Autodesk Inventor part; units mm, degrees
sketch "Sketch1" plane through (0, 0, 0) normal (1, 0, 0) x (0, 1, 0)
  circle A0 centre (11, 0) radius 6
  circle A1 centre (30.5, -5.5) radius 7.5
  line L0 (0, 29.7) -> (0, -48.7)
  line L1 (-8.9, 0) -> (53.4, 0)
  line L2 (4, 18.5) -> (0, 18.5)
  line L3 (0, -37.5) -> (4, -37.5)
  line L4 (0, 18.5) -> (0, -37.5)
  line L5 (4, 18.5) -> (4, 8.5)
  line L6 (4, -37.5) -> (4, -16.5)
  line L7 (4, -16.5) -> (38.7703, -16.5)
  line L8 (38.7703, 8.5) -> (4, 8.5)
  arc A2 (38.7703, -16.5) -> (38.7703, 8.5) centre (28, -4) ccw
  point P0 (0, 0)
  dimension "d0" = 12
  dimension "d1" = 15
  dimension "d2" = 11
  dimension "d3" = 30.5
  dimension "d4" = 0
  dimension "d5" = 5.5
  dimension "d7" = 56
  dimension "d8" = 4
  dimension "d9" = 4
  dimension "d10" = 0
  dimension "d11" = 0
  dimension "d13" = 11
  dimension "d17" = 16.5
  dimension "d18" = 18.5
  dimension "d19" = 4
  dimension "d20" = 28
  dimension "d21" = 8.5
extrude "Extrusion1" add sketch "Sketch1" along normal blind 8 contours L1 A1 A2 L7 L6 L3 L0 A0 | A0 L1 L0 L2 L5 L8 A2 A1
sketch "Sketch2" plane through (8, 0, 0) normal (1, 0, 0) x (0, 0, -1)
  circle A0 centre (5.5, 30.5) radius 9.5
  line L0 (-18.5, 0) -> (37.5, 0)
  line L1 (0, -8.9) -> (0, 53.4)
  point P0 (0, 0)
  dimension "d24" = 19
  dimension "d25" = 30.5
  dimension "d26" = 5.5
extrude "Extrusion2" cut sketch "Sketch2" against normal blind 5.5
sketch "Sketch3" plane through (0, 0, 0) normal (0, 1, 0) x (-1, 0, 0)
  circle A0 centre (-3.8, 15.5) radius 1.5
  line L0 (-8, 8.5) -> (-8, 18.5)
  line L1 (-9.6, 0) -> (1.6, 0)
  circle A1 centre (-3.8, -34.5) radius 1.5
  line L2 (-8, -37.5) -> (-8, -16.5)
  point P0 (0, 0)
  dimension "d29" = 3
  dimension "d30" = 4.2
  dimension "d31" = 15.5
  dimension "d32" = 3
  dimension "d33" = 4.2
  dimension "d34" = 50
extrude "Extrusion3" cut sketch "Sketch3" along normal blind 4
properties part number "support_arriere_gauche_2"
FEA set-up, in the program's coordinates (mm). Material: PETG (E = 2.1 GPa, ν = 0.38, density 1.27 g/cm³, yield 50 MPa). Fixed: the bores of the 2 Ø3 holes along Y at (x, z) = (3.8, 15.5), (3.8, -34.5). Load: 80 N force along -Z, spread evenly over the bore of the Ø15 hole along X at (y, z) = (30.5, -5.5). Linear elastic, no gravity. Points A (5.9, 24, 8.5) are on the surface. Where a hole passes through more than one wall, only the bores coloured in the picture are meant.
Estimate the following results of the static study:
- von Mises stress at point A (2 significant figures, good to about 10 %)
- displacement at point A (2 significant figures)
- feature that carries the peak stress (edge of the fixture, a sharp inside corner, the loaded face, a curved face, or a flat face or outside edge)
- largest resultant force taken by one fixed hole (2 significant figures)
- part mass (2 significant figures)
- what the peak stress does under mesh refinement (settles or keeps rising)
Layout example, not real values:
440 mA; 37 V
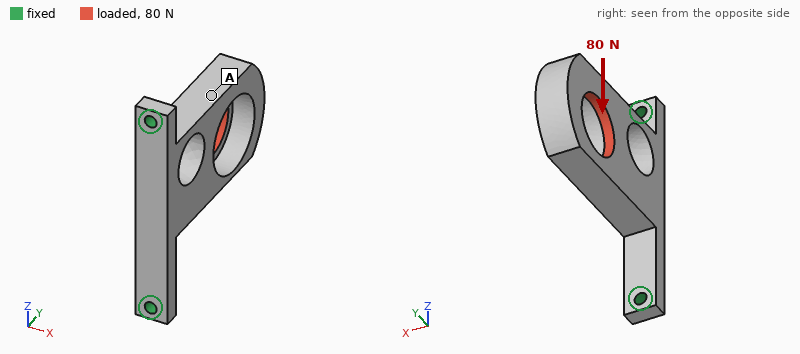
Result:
2.8 MPa; 0.36 mm; edge of the fixture; 72 N; 8.4 g; keeps rising
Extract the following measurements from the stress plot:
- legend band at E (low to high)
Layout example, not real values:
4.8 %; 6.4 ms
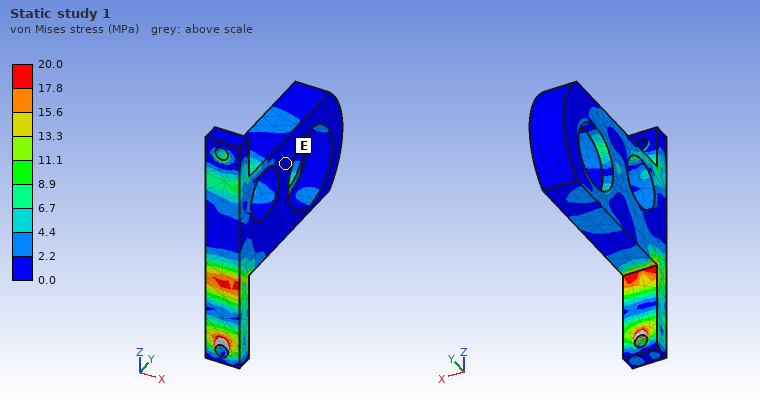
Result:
0.0 to 2.2 MPa
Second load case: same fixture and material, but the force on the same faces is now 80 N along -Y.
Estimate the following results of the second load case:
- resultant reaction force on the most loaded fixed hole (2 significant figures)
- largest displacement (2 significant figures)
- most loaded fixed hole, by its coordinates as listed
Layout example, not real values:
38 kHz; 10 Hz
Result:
49 N; 0.76 mm; (3.8, 15.5)
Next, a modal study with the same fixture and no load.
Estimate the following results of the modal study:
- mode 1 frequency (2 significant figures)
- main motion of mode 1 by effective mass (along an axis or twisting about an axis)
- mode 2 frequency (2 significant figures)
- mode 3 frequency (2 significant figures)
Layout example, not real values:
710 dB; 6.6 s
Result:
320 Hz; along X; 840 Hz; 1800 Hz
